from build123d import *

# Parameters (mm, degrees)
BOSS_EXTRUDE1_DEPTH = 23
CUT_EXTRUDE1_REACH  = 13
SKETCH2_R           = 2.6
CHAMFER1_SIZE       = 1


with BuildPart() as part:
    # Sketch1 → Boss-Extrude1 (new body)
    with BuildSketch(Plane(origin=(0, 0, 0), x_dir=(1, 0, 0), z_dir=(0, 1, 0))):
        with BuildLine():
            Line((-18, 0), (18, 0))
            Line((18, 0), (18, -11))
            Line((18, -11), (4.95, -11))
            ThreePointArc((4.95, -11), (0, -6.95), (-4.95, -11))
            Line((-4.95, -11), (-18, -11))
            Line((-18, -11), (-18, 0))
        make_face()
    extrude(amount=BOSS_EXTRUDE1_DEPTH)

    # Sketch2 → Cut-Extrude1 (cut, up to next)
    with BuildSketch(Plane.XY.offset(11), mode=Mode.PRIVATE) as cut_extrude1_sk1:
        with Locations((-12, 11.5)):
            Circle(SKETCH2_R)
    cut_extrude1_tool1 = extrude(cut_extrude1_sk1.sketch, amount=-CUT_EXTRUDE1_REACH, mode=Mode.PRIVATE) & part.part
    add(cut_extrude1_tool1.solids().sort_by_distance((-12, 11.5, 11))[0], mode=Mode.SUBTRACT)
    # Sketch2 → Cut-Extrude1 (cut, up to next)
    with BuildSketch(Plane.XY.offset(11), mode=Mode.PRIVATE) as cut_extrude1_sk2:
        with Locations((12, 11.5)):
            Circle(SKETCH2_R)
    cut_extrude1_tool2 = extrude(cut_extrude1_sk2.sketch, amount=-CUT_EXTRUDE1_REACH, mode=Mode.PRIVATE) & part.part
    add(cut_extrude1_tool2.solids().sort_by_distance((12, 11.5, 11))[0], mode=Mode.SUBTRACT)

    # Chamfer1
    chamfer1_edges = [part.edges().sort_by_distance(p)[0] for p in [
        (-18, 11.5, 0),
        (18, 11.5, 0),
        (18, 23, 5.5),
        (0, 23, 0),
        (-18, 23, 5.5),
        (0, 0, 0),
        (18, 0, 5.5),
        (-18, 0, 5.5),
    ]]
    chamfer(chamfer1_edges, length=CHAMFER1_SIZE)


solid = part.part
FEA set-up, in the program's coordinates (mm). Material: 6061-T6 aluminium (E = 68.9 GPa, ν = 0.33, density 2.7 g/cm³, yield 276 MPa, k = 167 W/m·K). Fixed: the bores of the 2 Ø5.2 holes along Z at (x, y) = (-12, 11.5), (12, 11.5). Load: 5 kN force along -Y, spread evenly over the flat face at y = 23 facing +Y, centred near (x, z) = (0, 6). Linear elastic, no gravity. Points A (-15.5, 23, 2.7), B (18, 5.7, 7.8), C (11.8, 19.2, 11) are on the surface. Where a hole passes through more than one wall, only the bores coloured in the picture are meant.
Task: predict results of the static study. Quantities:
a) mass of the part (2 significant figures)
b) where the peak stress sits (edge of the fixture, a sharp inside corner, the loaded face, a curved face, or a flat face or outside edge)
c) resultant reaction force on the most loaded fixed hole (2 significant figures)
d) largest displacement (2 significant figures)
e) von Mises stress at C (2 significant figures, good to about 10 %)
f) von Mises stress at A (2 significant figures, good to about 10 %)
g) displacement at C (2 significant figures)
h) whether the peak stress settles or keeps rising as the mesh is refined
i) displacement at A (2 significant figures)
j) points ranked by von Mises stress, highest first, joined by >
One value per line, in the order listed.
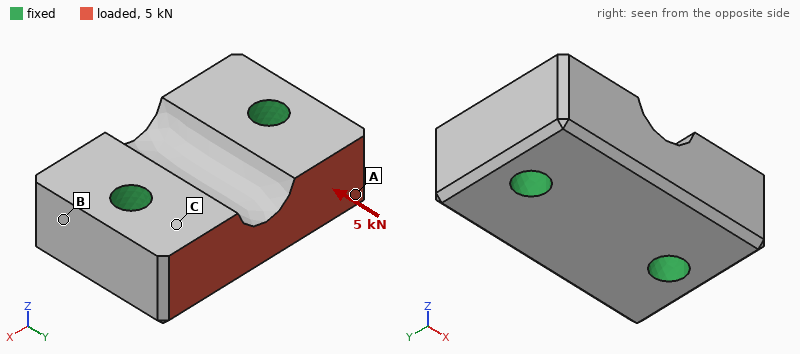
21 g
edge of the fixture
2.5 kN
3.8 µm
20 MPa
11 MPa
1.9 µm
keeps rising
1.9 µm
C > A > B
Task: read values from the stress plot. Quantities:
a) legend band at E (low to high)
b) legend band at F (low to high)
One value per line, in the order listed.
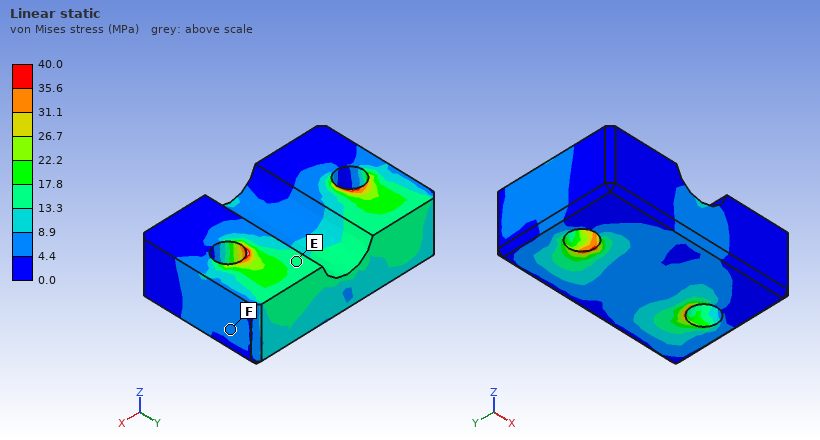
13.3 to 17.8 MPa
4.4 to 8.9 MPa
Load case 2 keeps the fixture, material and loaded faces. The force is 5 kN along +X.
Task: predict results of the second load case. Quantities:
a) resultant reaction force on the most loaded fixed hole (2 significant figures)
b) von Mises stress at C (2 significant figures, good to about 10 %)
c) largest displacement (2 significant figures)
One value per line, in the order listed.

3.1 kN
25 MPa
12 µm
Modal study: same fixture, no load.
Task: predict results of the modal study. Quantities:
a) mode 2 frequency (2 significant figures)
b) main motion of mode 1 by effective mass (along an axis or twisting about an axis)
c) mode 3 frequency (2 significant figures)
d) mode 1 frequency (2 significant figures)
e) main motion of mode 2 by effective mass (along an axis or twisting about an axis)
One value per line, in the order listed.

44 kHz
twisting about X
53 kHz
41 kHz
along Z
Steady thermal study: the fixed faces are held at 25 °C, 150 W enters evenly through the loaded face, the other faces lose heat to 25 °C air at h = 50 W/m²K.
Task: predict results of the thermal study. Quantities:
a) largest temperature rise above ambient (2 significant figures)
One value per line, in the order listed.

31 K
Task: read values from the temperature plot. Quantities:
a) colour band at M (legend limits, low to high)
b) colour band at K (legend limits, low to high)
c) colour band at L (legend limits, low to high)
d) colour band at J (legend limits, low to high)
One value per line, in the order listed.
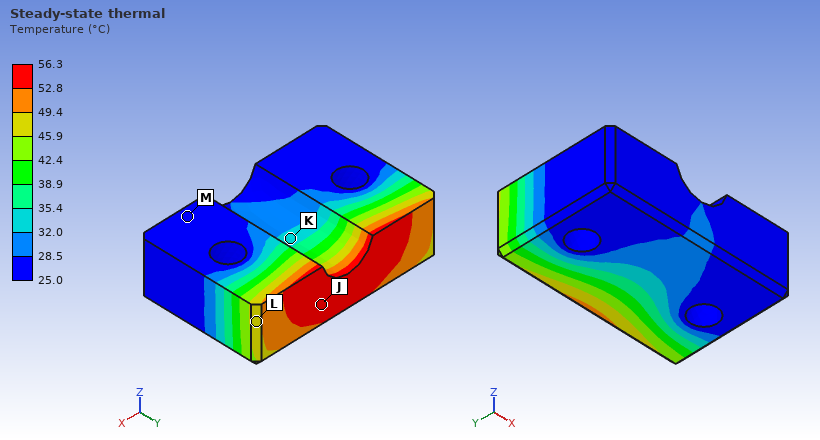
25.0 to 28.5 °C
32.0 to 35.4 °C
45.9 to 49.4 °C
52.8 to 56.3 °C
